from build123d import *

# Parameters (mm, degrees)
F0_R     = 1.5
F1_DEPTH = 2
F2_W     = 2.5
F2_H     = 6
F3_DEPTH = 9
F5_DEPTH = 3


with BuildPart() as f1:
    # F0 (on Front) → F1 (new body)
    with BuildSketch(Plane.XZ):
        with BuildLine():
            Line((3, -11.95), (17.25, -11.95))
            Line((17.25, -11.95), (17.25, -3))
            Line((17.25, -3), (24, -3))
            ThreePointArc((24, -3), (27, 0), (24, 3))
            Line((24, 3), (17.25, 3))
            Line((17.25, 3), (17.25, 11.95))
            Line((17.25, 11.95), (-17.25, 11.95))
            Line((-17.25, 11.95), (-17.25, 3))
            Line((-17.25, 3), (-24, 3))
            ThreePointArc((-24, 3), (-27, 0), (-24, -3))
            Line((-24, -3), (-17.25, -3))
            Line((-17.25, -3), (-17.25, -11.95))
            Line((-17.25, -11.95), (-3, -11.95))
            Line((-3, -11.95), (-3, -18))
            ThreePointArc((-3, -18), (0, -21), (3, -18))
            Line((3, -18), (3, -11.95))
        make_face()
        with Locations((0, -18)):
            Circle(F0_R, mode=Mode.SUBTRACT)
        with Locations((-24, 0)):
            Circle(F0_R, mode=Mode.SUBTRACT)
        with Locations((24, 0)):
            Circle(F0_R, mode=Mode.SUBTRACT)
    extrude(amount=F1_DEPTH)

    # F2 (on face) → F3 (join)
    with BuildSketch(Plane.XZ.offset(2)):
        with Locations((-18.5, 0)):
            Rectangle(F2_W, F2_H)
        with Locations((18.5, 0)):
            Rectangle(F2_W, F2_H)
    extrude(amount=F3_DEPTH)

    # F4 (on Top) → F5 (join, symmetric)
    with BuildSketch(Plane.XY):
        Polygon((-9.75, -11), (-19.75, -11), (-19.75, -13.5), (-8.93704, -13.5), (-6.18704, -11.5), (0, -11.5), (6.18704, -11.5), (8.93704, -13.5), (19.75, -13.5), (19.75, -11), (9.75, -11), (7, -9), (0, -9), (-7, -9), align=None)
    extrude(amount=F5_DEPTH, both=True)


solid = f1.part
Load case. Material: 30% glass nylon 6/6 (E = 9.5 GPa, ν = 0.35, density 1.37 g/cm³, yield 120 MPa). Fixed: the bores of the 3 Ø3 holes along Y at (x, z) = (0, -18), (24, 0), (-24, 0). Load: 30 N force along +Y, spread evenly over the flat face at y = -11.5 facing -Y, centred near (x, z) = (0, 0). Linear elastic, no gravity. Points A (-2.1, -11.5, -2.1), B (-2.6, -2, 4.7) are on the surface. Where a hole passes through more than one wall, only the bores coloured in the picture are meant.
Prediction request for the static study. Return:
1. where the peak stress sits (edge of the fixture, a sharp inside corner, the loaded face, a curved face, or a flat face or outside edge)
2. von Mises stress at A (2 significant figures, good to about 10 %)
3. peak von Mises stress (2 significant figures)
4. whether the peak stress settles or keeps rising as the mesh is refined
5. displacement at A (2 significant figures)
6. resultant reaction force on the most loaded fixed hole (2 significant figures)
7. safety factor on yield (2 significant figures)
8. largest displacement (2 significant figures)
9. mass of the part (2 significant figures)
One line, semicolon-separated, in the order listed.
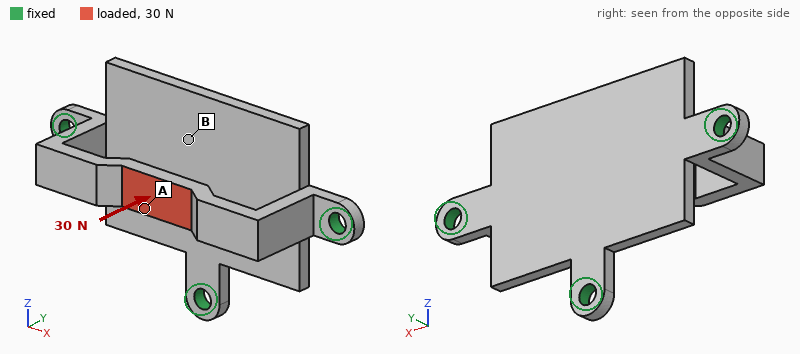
the loaded face; 21 MPa; 22 MPa; settles; 0.17 mm; 18 N; 5.4; 0.18 mm; 3.8 g
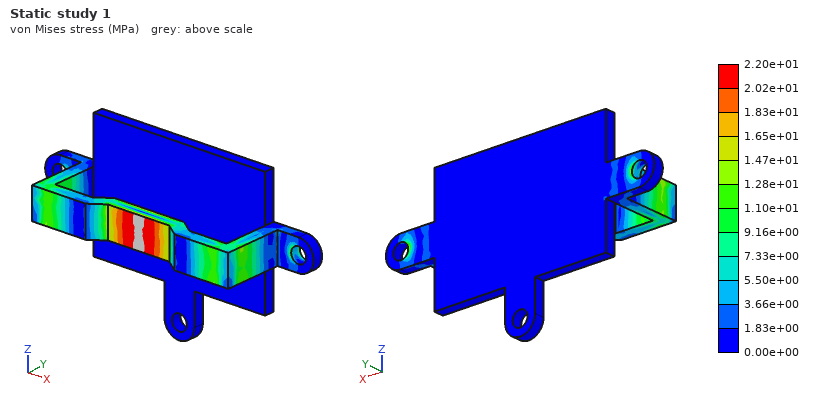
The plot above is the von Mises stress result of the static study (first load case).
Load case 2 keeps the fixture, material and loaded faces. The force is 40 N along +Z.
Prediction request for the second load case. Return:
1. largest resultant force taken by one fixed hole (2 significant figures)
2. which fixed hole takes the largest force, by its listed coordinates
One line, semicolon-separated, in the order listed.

22 N; (0, -18)
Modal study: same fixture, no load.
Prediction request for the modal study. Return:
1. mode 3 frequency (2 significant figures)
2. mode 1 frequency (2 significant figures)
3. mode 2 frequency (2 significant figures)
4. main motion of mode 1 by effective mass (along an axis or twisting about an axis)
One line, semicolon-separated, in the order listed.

3100 Hz; 2000 Hz; 3000 Hz; along Y
